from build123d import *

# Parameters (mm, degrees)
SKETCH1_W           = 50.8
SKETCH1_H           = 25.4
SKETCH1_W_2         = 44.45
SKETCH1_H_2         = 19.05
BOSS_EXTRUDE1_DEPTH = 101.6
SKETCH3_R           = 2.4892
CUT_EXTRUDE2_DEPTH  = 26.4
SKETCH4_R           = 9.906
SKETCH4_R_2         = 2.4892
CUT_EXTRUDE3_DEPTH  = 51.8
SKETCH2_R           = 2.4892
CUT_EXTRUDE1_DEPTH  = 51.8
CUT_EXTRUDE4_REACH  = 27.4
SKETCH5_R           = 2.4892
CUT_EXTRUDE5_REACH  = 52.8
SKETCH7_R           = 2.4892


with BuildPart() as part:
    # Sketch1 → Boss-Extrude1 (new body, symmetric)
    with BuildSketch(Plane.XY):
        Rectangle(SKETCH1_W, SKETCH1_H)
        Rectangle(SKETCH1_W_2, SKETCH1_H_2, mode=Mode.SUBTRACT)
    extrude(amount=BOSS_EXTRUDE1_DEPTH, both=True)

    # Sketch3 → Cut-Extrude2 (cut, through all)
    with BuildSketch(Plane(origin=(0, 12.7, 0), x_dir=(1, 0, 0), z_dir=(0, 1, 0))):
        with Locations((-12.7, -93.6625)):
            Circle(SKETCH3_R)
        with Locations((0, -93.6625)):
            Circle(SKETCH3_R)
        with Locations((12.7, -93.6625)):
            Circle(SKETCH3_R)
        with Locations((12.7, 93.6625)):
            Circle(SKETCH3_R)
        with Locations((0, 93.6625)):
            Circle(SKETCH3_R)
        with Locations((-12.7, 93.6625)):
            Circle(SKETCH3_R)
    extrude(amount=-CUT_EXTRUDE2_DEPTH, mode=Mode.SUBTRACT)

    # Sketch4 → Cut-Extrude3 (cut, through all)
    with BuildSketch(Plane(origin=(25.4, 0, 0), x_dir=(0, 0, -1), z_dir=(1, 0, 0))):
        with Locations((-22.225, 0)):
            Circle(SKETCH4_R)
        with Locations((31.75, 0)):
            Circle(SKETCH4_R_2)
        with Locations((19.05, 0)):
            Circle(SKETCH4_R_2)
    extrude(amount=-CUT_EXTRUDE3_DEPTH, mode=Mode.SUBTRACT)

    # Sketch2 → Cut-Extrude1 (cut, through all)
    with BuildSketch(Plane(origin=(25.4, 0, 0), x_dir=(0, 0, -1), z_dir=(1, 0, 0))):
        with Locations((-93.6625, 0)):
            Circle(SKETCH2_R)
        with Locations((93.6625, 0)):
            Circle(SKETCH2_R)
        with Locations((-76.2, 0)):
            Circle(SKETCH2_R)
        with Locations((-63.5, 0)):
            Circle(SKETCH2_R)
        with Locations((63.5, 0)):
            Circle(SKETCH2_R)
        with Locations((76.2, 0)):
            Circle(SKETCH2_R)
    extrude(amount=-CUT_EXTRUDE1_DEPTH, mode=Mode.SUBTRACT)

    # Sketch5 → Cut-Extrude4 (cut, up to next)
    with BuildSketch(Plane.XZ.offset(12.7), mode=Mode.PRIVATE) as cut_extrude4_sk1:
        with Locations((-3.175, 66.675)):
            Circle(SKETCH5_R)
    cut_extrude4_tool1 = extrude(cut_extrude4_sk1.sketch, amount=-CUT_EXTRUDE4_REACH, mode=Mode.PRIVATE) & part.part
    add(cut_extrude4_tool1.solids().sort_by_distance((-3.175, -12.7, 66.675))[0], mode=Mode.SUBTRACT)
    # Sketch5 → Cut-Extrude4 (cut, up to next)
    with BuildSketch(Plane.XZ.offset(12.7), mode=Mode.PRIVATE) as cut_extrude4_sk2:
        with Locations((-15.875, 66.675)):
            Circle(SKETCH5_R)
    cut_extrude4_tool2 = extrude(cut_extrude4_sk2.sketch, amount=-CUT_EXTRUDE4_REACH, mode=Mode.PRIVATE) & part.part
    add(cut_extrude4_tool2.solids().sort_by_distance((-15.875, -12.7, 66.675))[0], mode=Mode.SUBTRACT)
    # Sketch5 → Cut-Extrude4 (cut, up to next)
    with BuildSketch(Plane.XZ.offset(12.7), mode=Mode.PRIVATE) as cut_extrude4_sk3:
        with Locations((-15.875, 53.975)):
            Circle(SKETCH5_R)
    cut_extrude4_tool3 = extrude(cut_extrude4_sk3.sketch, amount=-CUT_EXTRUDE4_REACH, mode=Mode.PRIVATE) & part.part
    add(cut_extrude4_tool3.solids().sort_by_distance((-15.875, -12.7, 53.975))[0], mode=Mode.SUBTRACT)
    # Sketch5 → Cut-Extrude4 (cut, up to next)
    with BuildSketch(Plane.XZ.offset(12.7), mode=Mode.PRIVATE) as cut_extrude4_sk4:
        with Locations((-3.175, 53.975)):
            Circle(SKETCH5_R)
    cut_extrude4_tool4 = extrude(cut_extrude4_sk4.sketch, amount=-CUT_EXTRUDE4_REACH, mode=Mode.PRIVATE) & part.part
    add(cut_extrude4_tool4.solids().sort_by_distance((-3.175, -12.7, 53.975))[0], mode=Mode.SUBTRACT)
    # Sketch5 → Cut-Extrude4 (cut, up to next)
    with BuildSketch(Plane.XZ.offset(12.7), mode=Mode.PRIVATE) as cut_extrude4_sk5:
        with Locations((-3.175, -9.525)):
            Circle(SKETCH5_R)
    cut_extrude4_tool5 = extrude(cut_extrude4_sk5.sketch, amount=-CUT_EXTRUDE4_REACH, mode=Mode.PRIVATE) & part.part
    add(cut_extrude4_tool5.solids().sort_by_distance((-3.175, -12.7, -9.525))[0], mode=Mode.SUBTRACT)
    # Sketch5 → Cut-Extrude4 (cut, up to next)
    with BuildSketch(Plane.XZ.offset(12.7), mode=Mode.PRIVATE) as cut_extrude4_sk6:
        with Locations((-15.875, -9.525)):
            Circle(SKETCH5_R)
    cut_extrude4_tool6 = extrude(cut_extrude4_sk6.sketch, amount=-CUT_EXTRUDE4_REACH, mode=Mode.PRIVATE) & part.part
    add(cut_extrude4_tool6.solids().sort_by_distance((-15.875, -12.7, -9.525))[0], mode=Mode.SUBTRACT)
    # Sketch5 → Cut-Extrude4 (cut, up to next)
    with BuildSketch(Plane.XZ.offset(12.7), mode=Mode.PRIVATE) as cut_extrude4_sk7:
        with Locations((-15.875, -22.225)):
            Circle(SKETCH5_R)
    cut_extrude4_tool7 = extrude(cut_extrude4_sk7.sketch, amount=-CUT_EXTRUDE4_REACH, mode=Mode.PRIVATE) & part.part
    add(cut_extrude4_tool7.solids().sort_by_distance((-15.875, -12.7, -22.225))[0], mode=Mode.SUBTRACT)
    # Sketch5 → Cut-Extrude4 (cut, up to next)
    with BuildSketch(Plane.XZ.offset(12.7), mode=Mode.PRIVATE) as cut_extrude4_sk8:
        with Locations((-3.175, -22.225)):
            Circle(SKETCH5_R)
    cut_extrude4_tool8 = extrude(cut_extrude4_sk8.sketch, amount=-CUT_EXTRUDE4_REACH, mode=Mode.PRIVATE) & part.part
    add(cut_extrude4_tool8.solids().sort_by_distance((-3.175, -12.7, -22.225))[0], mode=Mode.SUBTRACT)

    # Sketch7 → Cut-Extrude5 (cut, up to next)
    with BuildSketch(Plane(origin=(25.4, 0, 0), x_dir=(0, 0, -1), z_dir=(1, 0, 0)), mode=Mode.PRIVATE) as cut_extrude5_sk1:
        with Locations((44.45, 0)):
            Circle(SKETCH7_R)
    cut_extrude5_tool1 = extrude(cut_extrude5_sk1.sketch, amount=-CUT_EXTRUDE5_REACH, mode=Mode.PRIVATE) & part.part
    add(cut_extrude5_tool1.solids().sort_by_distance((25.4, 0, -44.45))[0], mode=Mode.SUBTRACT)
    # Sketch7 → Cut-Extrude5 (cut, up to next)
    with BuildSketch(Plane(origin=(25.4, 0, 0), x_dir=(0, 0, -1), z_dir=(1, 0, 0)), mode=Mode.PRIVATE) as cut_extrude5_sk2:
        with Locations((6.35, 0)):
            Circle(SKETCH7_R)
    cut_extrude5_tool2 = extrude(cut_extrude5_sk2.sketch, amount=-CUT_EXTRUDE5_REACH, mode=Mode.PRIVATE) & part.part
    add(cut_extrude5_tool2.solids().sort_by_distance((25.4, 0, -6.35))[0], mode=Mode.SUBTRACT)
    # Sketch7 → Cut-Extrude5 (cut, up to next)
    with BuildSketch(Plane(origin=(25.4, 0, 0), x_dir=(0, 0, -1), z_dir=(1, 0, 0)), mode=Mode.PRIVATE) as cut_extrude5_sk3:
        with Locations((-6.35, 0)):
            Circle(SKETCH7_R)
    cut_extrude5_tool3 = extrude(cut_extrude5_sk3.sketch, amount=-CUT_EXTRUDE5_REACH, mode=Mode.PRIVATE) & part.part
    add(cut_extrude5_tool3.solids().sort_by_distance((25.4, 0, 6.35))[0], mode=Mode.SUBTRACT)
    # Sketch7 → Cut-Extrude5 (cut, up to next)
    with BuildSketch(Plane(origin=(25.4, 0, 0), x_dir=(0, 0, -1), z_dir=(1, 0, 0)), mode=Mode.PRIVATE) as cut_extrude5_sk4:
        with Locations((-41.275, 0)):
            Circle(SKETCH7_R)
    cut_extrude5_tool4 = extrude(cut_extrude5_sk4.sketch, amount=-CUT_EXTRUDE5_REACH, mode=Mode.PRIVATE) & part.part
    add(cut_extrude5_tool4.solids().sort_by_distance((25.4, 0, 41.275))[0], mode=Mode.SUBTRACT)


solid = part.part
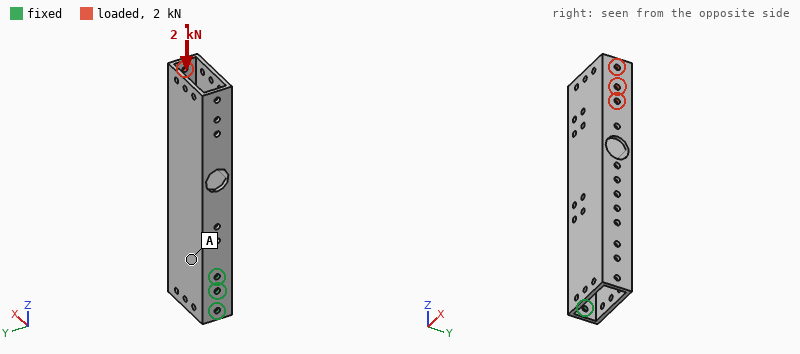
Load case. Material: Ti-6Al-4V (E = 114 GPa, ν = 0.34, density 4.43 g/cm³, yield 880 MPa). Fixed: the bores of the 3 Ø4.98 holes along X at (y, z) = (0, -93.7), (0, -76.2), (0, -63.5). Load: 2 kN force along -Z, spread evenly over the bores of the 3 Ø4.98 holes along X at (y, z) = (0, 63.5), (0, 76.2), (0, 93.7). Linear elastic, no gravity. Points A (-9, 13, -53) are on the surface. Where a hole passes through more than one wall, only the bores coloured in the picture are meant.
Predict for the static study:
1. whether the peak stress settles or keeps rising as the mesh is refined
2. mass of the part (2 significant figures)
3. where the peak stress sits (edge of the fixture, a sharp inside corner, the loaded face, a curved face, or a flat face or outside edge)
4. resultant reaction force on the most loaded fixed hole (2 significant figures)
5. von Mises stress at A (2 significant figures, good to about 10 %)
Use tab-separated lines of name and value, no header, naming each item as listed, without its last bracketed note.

whether the peak stress settles or keeps rising as the mesh is refined	keeps rising
mass of the part	380 g
where the peak stress sits	edge of the fixture
resultant reaction force on the most loaded fixed hole	2.9 kN
von Mises stress at A	19 MPa
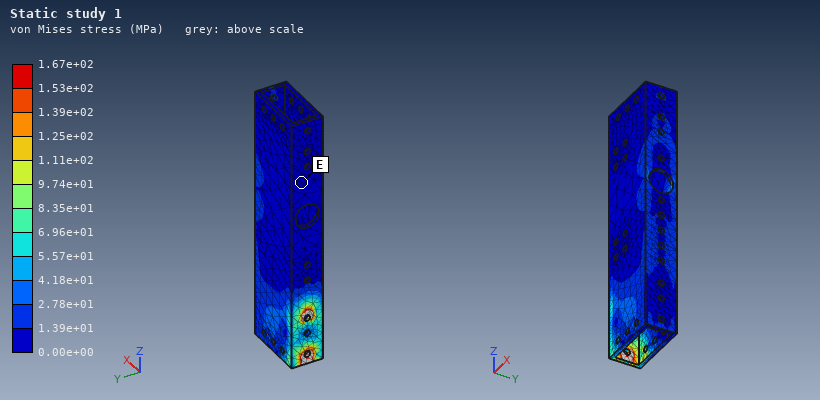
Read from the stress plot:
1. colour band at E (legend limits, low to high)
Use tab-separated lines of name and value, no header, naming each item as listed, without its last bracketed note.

colour band at E	0.00e+00 to 1.39e+01 MPa
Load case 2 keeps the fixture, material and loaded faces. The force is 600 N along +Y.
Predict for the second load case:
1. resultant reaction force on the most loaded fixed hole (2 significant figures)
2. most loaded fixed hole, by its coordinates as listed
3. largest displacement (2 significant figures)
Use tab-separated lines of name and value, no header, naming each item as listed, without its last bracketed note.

resultant reaction force on the most loaded fixed hole	3.2 kN
most loaded fixed hole, by its coordinates as listed	(0, -63.5)
largest displacement	0.70 mm
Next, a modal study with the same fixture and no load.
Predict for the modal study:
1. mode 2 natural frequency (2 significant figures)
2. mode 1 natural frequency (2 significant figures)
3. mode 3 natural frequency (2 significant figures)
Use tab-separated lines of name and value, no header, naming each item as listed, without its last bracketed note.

mode 2 natural frequency	460 Hz
mode 1 natural frequency	450 Hz
mode 3 natural frequency	780 Hz
